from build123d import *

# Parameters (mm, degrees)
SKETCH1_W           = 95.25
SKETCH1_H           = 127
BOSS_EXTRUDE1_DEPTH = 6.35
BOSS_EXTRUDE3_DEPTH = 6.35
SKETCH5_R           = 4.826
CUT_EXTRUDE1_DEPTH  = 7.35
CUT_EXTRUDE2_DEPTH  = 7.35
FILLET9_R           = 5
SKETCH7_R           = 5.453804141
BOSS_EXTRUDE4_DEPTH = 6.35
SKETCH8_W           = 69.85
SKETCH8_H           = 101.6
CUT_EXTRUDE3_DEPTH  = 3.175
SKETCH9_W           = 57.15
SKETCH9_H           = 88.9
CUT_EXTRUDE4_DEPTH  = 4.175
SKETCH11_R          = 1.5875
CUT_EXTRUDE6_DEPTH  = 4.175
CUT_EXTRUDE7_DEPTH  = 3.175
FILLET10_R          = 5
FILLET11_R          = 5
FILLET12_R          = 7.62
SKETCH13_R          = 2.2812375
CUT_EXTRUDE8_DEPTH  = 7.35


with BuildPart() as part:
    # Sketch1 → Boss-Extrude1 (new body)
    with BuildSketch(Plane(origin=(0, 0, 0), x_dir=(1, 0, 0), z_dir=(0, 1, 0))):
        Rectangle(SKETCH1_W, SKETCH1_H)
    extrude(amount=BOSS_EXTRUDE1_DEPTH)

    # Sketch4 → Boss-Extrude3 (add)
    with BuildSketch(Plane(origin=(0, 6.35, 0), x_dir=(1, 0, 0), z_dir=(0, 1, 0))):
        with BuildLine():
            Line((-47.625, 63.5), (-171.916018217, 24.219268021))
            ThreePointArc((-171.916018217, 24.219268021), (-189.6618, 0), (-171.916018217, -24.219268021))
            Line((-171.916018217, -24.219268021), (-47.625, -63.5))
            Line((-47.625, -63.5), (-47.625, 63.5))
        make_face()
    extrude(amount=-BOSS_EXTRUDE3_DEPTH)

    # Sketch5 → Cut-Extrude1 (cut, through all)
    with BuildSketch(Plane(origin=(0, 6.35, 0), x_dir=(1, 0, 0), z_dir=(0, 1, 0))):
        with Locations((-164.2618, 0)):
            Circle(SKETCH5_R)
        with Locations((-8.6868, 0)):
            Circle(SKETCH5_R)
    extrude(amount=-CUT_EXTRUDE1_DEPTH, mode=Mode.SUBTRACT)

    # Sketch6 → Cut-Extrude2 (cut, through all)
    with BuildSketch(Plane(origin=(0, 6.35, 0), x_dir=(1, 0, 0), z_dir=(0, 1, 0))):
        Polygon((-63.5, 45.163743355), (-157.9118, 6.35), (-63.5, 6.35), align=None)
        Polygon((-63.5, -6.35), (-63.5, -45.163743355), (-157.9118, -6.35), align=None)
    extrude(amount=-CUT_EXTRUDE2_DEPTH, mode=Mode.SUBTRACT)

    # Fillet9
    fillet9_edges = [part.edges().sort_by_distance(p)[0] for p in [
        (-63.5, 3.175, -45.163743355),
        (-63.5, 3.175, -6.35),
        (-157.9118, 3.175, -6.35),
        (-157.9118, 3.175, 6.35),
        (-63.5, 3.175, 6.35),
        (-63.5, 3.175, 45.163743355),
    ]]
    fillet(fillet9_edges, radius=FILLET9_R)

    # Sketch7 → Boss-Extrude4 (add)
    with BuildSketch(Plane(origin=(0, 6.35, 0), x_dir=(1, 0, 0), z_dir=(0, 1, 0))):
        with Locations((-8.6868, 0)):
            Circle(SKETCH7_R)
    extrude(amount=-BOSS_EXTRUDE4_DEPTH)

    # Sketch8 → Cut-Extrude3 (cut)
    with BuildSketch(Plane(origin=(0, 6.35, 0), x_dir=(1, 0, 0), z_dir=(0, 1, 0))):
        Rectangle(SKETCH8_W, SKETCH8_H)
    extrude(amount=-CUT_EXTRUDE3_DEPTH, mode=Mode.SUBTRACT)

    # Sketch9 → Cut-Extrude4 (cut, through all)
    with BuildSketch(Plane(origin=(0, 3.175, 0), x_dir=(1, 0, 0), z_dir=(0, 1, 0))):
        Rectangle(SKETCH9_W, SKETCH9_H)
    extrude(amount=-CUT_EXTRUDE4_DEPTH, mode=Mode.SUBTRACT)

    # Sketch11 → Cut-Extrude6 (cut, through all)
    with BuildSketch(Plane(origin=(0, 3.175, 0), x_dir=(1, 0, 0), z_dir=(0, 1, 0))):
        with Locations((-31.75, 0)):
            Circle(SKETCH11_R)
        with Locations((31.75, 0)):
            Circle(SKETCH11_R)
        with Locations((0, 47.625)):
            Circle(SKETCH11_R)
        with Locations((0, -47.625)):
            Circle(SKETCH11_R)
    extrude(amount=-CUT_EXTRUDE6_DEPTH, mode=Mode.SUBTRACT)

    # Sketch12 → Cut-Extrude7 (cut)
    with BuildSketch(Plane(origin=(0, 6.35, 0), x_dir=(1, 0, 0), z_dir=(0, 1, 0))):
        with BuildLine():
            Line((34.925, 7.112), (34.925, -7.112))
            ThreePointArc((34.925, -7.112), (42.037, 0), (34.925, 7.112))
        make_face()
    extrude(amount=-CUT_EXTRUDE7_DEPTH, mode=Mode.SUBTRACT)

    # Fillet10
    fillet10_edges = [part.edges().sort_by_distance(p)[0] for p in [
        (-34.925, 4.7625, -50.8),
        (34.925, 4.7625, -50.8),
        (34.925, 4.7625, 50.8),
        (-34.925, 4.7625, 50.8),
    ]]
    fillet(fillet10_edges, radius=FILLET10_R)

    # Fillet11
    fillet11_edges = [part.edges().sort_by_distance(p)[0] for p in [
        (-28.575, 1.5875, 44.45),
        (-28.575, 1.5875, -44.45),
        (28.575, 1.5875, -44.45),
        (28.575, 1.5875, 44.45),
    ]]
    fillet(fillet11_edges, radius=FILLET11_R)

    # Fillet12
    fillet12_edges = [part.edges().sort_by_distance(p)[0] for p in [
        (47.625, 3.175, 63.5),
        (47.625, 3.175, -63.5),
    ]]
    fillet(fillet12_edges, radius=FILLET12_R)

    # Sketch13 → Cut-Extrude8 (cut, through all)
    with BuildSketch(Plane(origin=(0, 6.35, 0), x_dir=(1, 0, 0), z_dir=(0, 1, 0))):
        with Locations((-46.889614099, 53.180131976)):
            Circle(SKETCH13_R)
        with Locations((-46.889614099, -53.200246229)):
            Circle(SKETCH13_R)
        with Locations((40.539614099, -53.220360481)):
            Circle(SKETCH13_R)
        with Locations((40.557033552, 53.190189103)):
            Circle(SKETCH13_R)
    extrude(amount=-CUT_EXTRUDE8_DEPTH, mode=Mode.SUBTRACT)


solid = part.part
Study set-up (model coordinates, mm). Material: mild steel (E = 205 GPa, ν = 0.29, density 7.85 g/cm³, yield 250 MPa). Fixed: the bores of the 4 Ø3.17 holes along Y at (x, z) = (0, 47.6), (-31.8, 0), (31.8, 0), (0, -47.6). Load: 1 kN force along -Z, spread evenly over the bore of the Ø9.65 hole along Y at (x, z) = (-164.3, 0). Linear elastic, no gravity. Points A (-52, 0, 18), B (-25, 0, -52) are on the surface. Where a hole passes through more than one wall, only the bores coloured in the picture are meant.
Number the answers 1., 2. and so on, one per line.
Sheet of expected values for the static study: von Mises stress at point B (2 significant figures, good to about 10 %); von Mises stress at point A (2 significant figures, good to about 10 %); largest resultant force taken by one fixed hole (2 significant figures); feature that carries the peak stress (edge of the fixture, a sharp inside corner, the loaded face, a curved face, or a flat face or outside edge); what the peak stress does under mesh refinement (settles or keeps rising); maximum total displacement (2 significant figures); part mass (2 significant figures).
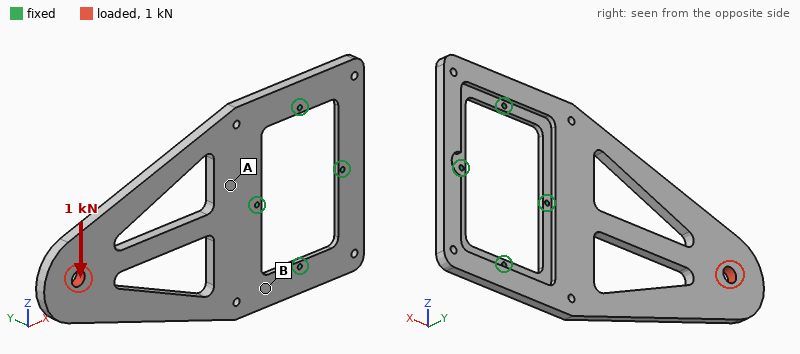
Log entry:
1. 12 MPa
2. 5.2 MPa
3. 1.2 kN
4. edge of the fixture
5. keeps rising
6. 32 µm
7. 690 g
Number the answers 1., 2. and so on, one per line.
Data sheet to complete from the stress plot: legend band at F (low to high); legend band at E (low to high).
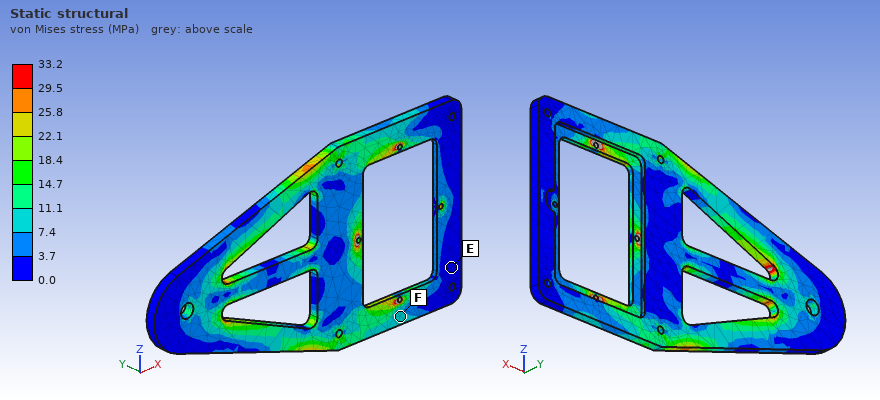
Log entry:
1. 7.4 to 11.1 MPa
2. 0.0 to 3.7 MPa
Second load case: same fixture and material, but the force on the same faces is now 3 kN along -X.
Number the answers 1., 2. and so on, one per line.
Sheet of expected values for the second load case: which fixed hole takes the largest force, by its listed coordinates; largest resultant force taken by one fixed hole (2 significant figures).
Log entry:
1. (-31.8, 0)
2. 1.2 kN
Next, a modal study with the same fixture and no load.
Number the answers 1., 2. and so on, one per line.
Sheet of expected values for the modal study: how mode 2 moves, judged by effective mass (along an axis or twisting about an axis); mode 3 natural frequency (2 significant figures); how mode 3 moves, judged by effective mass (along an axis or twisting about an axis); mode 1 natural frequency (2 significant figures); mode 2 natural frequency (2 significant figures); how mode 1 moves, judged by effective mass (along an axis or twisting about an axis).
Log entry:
1. twisting about X
2. 960 Hz
3. along Y
4. 170 Hz
5. 700 Hz
6. along Y
